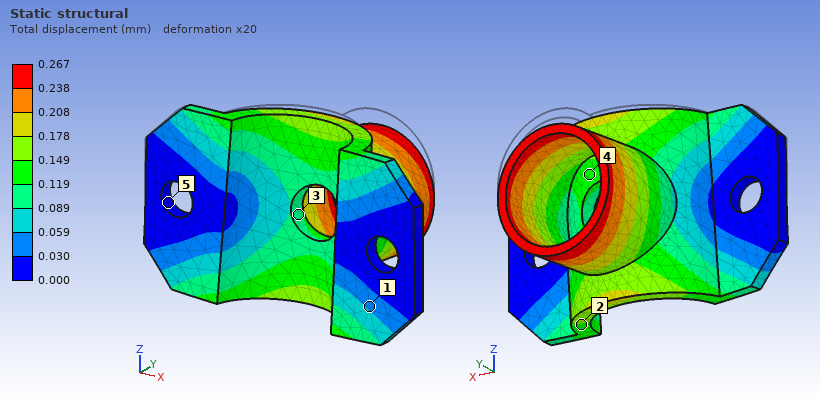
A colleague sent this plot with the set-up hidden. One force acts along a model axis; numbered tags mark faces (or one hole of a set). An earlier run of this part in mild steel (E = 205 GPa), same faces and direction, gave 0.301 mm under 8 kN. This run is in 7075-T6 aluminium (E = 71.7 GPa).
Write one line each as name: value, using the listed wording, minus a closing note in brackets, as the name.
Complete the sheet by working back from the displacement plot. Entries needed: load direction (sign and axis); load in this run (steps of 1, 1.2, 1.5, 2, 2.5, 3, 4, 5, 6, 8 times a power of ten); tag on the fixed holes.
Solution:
load direction: -Z
load in this run: 2.5 kN
tag on the fixed holes: 5
